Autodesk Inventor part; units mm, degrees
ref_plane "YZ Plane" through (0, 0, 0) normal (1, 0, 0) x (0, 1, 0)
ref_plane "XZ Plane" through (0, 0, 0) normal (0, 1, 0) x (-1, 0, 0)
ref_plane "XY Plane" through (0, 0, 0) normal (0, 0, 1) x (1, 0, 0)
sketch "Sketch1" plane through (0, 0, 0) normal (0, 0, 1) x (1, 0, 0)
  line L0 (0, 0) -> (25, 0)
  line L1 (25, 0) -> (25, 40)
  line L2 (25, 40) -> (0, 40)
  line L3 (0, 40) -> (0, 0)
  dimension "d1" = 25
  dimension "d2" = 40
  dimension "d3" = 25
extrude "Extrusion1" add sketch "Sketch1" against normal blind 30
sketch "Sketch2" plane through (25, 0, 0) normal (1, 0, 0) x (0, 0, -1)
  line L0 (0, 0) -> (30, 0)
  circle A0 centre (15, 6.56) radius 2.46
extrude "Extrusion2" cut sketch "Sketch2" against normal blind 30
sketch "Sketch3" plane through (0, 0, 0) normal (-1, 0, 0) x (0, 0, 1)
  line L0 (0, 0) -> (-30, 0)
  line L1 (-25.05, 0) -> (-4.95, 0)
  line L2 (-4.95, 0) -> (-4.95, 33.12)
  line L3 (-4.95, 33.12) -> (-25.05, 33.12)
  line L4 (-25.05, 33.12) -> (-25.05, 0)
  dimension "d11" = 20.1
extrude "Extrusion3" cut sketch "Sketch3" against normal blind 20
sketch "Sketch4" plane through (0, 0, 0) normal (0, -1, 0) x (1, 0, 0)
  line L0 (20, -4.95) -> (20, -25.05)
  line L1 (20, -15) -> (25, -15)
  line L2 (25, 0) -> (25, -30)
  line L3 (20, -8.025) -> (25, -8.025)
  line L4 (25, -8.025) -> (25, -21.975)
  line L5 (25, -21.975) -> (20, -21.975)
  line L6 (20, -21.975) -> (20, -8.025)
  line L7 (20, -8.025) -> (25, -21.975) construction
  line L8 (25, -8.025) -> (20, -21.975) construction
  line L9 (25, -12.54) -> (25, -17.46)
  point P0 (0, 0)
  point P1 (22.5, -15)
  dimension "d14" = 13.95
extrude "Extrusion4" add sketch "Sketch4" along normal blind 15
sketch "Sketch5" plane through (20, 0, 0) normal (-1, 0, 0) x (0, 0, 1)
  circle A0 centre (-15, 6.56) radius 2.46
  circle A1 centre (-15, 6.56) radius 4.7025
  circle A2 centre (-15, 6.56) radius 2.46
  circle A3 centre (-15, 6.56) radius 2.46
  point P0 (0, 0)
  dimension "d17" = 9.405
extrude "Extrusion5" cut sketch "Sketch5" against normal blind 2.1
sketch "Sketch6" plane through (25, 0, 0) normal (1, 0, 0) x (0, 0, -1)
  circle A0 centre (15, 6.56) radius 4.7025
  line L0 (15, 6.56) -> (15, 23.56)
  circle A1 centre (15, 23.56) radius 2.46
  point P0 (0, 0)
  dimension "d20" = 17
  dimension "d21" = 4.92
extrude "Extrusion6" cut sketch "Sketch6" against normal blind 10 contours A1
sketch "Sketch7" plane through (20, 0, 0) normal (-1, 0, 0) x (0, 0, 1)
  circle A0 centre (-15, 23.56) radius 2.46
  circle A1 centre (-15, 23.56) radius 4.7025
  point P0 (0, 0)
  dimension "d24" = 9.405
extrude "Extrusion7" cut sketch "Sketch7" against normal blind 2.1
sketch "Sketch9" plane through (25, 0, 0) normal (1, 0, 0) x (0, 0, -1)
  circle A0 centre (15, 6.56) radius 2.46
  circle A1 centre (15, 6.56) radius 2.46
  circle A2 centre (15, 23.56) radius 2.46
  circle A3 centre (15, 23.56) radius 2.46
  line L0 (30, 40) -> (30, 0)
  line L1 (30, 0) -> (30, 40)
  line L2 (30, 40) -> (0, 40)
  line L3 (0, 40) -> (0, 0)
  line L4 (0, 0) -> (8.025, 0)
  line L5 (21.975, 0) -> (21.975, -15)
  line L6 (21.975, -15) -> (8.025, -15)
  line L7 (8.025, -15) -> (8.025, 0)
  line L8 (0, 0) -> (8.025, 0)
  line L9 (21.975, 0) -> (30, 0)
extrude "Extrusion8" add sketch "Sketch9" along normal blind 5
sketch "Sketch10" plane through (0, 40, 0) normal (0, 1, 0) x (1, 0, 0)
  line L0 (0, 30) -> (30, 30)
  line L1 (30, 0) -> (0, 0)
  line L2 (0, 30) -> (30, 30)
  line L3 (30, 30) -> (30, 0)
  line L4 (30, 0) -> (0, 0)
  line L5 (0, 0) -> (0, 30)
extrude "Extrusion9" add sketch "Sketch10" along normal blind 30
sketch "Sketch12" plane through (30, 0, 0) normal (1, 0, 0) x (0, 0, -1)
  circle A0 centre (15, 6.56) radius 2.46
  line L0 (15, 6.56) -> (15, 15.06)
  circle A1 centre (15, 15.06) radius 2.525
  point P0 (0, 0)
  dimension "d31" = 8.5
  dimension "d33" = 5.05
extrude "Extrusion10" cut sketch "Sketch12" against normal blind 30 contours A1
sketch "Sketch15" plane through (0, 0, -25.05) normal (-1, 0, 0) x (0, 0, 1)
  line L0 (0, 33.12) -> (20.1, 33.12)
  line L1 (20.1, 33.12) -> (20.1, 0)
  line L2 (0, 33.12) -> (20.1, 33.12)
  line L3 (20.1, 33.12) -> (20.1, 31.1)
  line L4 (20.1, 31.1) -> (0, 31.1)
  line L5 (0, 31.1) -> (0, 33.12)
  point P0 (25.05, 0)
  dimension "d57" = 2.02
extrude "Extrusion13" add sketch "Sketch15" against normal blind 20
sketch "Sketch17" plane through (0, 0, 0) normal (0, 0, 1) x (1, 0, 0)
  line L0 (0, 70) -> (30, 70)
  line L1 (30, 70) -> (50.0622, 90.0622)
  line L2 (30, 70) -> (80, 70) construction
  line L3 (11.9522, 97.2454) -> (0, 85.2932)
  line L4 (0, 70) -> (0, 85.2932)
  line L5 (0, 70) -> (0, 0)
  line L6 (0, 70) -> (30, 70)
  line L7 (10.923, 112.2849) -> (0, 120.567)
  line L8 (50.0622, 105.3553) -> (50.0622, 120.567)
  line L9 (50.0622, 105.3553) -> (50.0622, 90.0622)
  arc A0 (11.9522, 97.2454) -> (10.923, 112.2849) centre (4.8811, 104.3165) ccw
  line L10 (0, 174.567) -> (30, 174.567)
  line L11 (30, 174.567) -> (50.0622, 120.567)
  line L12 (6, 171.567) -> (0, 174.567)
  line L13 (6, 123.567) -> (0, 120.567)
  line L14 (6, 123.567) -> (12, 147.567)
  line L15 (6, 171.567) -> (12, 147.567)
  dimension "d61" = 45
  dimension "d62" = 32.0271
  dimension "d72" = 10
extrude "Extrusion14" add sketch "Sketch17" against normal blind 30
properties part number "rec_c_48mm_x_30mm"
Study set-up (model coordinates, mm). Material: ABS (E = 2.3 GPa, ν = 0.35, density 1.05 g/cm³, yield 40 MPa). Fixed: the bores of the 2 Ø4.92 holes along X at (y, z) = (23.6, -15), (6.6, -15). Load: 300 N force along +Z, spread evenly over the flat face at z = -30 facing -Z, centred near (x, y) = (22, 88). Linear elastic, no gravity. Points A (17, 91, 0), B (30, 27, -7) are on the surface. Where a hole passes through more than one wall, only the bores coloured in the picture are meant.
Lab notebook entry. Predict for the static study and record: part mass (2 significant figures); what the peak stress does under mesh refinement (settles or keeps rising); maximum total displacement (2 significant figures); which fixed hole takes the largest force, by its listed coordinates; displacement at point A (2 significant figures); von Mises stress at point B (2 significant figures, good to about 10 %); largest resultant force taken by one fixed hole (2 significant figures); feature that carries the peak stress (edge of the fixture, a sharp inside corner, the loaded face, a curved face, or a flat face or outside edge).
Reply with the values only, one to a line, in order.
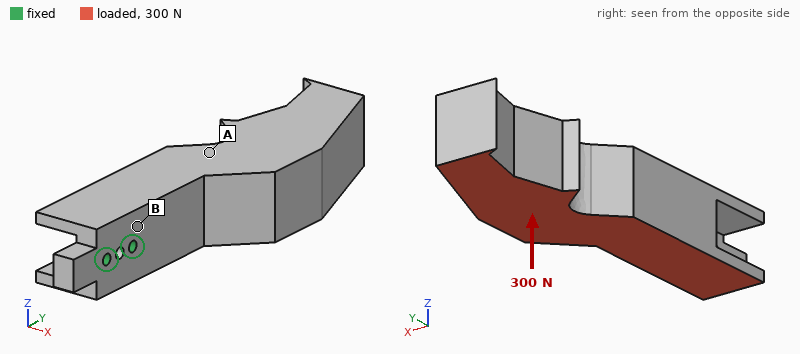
170 g
keeps rising
2.0 mm
(23.6, -15)
0.81 mm
5.6 MPa
1.1 kN
edge of the fixture
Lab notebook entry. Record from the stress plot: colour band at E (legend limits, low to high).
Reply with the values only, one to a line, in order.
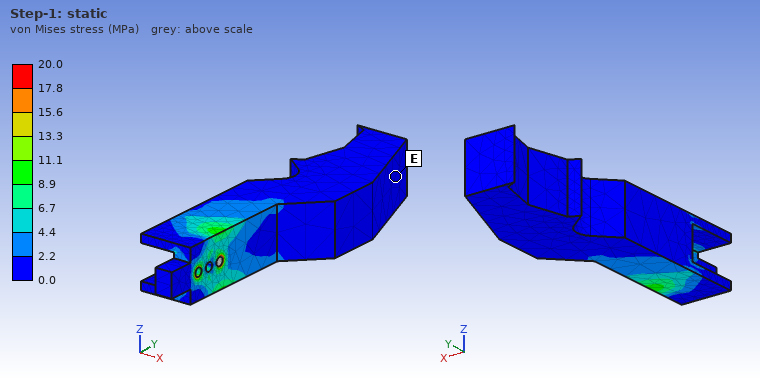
0.0 to 2.2 MPa
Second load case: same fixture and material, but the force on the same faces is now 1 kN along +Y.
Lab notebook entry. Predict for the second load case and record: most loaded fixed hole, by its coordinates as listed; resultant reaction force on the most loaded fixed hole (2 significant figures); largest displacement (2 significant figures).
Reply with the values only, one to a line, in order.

(23.6, -15)
970 N
1.7 mm
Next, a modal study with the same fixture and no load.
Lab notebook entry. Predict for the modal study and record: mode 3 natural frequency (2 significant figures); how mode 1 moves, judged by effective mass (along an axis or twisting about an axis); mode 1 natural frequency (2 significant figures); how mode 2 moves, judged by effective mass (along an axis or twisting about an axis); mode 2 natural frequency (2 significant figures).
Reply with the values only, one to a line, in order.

630 Hz
along X
160 Hz
along Z
180 Hz
